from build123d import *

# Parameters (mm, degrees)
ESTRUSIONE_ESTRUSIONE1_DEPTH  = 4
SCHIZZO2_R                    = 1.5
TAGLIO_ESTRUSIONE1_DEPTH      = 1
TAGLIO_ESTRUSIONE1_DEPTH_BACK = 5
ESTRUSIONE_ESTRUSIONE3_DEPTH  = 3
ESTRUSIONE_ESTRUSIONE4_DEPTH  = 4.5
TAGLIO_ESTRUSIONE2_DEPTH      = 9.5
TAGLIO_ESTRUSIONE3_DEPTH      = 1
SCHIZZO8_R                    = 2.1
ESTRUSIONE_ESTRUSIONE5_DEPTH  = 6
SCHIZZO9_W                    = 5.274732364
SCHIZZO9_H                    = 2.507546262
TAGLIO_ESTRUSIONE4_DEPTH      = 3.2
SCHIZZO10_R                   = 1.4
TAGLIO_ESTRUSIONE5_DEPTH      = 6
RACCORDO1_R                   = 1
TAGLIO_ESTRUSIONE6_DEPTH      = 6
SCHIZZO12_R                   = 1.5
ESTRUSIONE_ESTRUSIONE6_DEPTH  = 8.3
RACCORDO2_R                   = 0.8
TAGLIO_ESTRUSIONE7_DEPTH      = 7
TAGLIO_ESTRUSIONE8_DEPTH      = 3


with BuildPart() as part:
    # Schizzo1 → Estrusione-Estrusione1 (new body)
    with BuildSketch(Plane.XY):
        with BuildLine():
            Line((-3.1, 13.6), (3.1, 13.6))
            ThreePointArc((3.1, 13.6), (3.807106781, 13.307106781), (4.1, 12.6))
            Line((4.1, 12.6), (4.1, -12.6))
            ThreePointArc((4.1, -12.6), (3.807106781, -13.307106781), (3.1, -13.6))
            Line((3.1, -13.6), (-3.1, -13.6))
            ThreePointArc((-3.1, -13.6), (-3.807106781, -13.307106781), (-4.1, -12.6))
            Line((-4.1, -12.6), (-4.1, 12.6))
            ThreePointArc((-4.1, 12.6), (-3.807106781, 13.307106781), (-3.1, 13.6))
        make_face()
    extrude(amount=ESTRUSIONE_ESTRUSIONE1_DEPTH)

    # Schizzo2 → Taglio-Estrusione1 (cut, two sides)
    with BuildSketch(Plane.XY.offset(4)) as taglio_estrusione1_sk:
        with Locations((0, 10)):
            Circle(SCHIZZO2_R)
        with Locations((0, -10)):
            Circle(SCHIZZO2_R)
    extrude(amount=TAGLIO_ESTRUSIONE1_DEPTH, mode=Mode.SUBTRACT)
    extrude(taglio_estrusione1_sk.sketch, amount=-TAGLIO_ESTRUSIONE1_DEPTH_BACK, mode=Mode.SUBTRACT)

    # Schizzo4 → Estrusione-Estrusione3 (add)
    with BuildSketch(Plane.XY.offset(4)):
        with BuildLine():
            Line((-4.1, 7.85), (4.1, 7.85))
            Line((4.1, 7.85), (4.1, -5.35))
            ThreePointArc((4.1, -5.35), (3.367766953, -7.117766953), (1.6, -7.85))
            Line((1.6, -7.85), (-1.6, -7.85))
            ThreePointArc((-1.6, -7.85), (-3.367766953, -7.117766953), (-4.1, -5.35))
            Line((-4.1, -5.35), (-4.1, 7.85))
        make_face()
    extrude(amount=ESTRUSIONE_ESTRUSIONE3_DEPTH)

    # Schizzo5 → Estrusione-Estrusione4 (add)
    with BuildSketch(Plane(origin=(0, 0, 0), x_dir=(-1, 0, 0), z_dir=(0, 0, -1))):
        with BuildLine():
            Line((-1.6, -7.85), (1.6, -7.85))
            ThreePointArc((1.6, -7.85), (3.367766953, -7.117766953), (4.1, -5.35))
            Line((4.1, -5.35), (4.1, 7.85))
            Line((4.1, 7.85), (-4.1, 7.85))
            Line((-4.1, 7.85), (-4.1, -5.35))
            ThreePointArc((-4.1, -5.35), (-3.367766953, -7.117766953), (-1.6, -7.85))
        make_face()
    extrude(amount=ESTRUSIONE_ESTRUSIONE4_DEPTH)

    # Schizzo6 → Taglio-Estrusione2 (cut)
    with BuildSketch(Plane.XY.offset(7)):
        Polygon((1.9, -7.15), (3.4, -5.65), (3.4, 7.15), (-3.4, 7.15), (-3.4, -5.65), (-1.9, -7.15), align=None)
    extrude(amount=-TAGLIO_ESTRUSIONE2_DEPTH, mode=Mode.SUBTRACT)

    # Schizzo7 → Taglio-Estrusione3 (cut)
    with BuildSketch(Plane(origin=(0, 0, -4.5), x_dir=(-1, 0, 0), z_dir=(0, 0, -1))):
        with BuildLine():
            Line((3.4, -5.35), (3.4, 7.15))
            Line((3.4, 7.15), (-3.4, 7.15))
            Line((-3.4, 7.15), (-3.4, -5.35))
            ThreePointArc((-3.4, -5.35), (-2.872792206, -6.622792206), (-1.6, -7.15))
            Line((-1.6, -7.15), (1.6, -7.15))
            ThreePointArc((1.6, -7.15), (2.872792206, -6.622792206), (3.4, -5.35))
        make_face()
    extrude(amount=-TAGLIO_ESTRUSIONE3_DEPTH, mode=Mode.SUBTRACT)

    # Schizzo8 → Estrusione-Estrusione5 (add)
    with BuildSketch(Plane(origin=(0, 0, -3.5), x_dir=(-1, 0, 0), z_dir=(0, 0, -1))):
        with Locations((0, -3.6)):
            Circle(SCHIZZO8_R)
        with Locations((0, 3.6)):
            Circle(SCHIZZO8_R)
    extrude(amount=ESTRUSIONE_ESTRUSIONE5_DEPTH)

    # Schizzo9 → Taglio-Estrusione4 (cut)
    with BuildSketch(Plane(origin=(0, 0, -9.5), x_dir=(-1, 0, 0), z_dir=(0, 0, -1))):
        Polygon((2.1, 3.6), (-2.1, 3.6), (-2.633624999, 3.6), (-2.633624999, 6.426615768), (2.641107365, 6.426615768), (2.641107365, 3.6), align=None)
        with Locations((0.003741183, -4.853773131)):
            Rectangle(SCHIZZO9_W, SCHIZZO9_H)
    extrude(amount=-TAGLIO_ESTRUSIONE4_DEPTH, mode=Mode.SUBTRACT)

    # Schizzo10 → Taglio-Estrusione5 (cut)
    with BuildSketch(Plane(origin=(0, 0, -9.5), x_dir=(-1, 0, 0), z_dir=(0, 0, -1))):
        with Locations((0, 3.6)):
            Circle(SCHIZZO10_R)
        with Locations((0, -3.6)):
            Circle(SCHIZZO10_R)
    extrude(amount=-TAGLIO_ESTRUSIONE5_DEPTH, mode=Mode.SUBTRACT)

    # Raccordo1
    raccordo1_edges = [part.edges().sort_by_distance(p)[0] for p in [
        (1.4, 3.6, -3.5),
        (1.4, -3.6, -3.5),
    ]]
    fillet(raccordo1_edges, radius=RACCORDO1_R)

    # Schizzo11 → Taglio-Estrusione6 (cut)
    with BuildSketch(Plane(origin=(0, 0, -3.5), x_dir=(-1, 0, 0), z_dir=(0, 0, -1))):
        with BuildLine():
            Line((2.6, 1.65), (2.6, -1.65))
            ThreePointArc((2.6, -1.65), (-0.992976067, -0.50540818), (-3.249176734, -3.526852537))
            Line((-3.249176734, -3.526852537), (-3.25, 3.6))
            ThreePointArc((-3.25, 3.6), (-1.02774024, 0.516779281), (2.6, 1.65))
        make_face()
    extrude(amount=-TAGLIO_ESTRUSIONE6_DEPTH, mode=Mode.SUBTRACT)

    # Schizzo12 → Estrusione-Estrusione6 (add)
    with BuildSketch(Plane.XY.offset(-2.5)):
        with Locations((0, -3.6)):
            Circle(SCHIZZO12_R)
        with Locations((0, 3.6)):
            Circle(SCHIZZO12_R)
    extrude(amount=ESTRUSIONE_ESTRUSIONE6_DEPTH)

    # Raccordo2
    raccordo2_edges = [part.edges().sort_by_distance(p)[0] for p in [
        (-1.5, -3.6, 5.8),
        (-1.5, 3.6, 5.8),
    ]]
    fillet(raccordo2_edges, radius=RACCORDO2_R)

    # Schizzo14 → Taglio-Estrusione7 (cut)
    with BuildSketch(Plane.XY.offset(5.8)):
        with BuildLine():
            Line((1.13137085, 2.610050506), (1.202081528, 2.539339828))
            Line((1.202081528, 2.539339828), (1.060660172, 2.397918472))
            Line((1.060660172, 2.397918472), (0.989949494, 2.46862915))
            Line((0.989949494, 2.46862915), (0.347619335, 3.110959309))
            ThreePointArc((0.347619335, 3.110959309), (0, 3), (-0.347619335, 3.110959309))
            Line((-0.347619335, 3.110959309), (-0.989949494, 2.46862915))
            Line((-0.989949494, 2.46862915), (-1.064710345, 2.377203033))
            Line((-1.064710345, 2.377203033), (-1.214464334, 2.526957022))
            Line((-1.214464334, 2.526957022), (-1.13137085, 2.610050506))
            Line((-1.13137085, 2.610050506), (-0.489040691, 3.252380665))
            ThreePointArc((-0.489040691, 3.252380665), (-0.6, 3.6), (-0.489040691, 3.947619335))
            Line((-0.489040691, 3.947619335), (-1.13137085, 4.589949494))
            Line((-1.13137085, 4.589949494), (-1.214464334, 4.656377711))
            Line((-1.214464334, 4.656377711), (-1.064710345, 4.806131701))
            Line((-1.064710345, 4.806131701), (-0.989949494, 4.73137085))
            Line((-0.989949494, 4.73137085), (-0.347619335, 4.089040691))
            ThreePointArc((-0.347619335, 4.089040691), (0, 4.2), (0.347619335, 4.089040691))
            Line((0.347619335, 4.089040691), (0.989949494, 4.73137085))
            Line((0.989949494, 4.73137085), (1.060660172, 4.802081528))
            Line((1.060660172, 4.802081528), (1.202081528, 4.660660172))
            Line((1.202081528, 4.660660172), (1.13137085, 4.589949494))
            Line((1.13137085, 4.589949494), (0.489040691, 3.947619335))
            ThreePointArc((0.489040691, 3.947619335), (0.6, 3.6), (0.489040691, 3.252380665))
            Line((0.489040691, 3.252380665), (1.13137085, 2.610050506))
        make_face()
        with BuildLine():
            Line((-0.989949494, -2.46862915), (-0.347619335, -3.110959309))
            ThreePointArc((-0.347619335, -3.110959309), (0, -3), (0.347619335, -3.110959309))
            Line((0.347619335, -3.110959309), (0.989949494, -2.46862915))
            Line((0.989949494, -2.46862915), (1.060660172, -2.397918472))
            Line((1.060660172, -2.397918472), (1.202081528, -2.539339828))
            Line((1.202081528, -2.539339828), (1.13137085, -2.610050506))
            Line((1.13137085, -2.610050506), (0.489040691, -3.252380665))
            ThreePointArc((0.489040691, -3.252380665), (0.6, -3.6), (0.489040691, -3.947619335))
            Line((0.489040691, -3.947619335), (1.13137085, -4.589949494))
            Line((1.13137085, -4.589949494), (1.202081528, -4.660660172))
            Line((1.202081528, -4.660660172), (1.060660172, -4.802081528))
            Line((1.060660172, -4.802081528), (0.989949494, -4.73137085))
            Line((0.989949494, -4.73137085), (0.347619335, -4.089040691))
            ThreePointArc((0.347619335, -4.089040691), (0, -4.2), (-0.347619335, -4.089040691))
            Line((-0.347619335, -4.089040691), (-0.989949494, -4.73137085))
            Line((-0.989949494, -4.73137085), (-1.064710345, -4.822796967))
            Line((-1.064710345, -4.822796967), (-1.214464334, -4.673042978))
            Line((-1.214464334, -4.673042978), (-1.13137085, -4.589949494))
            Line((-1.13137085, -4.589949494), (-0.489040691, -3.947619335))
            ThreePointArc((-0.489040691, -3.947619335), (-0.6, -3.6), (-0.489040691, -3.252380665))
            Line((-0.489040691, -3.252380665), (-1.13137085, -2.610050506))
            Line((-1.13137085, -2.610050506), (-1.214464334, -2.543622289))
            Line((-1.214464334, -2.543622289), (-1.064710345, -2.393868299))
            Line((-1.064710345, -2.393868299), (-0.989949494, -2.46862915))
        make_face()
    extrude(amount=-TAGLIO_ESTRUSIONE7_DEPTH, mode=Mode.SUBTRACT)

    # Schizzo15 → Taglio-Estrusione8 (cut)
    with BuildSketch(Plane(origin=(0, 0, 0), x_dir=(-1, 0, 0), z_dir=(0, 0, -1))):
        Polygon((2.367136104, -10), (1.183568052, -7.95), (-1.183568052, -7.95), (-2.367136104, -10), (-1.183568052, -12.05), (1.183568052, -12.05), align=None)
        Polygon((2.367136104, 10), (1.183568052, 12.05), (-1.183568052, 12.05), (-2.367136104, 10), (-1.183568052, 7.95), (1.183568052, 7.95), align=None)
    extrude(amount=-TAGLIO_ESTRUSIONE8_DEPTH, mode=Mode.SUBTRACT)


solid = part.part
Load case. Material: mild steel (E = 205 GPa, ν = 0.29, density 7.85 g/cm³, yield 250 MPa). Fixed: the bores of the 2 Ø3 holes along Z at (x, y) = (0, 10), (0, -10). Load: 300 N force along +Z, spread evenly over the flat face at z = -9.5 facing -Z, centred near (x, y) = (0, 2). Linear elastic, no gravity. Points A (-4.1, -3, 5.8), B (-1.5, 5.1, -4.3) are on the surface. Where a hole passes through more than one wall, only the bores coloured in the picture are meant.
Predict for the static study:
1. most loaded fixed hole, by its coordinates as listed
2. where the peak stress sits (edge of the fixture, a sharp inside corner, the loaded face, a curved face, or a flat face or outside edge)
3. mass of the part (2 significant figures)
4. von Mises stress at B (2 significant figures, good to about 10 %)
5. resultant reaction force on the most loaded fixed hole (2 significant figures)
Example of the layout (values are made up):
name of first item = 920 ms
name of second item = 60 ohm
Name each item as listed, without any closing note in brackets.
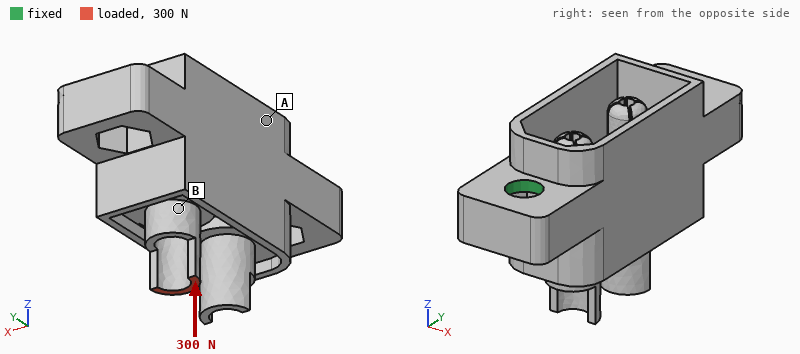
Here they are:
most loaded fixed hole, by its coordinates as listed = (0, 10)
where the peak stress sits = a flat face or outside edge
mass of the part = 6.9 g
von Mises stress at B = 49 MPa
resultant reaction force on the most loaded fixed hole = 200 N
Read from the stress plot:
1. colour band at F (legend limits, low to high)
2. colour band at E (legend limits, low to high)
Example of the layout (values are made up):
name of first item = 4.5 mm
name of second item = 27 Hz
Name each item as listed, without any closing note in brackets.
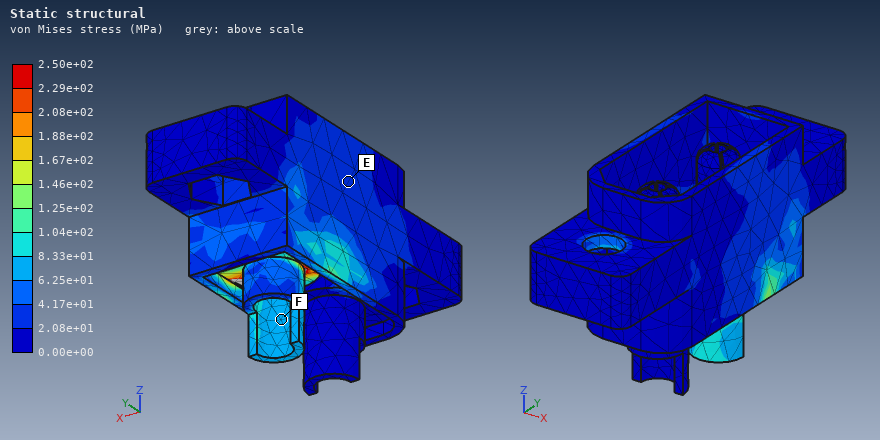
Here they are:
colour band at F = 6.25e+01 to 8.33e+01 MPa
colour band at E = 2.08e+01 to 4.17e+01 MPa
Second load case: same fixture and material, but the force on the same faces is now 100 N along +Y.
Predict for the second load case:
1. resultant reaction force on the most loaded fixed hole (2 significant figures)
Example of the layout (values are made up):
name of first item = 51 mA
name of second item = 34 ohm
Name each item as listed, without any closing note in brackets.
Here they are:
resultant reaction force on the most loaded fixed hole = 89 N
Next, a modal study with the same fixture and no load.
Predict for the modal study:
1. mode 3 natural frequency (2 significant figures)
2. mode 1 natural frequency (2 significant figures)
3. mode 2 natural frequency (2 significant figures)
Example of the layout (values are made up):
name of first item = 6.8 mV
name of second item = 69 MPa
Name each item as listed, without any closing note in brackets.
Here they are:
mode 3 natural frequency = 12 kHz
mode 1 natural frequency = 12 kHz
mode 2 natural frequency = 12 kHz
